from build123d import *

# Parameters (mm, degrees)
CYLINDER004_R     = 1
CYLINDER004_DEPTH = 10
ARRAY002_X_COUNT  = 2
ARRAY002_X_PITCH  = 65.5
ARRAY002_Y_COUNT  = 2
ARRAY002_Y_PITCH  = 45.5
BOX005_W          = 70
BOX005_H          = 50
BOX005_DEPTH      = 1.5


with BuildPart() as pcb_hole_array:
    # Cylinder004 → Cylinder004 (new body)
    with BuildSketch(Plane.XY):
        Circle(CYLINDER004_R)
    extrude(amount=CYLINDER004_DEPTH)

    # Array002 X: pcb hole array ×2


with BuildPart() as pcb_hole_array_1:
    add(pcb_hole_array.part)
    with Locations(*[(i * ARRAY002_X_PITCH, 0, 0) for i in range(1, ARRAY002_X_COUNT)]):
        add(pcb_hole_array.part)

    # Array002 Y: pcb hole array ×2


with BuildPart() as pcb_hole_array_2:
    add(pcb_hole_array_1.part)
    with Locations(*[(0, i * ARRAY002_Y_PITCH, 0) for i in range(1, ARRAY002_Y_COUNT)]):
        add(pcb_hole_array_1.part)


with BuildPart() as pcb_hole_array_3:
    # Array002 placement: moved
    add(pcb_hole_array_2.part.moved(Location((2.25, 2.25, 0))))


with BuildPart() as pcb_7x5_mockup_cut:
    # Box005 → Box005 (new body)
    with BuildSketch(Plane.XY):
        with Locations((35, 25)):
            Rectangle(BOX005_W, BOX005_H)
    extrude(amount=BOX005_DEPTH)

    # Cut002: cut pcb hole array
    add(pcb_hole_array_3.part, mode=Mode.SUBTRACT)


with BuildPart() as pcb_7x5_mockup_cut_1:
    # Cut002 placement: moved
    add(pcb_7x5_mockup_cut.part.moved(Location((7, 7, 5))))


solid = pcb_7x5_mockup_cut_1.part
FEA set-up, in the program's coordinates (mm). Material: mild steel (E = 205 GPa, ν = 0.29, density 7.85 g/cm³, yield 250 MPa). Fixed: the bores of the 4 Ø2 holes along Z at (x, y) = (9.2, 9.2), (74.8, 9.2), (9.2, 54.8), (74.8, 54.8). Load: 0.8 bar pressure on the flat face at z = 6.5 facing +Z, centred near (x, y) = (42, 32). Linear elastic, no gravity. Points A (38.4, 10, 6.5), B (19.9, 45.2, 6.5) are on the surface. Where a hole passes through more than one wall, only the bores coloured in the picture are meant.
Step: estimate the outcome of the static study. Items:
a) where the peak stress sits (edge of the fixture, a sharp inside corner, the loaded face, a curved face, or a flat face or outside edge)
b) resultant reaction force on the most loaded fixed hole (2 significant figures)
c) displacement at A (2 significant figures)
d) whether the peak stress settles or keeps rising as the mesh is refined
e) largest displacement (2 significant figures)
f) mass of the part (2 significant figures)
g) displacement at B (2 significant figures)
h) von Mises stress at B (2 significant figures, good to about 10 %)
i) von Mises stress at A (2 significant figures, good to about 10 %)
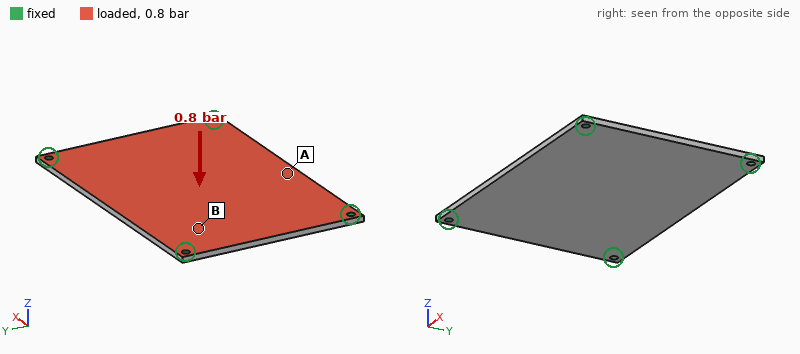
edge of the fixture
70 N
0.11 mm
keeps rising
0.13 mm
41 g
0.056 mm
17 MPa
54 MPa
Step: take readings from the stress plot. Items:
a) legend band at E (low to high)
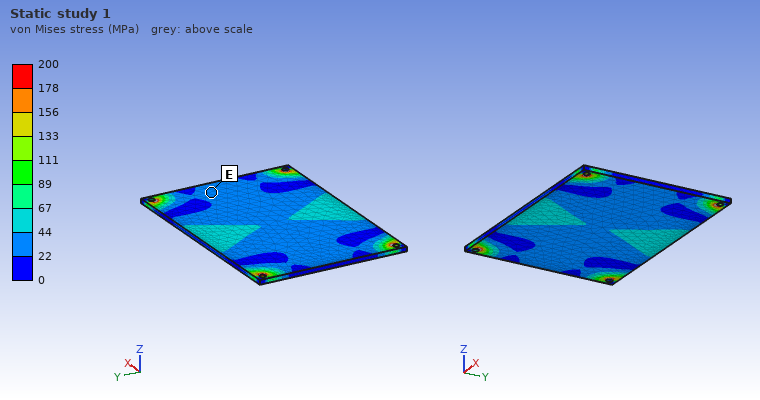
22 to 44 MPa
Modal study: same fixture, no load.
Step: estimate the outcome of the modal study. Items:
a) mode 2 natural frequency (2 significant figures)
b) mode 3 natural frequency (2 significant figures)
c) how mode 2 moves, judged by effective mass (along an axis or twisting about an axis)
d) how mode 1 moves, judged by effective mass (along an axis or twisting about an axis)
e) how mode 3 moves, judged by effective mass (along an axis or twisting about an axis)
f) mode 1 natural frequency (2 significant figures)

2400 Hz
3300 Hz
twisting about X
along Z
twisting about Y
1400 Hz
